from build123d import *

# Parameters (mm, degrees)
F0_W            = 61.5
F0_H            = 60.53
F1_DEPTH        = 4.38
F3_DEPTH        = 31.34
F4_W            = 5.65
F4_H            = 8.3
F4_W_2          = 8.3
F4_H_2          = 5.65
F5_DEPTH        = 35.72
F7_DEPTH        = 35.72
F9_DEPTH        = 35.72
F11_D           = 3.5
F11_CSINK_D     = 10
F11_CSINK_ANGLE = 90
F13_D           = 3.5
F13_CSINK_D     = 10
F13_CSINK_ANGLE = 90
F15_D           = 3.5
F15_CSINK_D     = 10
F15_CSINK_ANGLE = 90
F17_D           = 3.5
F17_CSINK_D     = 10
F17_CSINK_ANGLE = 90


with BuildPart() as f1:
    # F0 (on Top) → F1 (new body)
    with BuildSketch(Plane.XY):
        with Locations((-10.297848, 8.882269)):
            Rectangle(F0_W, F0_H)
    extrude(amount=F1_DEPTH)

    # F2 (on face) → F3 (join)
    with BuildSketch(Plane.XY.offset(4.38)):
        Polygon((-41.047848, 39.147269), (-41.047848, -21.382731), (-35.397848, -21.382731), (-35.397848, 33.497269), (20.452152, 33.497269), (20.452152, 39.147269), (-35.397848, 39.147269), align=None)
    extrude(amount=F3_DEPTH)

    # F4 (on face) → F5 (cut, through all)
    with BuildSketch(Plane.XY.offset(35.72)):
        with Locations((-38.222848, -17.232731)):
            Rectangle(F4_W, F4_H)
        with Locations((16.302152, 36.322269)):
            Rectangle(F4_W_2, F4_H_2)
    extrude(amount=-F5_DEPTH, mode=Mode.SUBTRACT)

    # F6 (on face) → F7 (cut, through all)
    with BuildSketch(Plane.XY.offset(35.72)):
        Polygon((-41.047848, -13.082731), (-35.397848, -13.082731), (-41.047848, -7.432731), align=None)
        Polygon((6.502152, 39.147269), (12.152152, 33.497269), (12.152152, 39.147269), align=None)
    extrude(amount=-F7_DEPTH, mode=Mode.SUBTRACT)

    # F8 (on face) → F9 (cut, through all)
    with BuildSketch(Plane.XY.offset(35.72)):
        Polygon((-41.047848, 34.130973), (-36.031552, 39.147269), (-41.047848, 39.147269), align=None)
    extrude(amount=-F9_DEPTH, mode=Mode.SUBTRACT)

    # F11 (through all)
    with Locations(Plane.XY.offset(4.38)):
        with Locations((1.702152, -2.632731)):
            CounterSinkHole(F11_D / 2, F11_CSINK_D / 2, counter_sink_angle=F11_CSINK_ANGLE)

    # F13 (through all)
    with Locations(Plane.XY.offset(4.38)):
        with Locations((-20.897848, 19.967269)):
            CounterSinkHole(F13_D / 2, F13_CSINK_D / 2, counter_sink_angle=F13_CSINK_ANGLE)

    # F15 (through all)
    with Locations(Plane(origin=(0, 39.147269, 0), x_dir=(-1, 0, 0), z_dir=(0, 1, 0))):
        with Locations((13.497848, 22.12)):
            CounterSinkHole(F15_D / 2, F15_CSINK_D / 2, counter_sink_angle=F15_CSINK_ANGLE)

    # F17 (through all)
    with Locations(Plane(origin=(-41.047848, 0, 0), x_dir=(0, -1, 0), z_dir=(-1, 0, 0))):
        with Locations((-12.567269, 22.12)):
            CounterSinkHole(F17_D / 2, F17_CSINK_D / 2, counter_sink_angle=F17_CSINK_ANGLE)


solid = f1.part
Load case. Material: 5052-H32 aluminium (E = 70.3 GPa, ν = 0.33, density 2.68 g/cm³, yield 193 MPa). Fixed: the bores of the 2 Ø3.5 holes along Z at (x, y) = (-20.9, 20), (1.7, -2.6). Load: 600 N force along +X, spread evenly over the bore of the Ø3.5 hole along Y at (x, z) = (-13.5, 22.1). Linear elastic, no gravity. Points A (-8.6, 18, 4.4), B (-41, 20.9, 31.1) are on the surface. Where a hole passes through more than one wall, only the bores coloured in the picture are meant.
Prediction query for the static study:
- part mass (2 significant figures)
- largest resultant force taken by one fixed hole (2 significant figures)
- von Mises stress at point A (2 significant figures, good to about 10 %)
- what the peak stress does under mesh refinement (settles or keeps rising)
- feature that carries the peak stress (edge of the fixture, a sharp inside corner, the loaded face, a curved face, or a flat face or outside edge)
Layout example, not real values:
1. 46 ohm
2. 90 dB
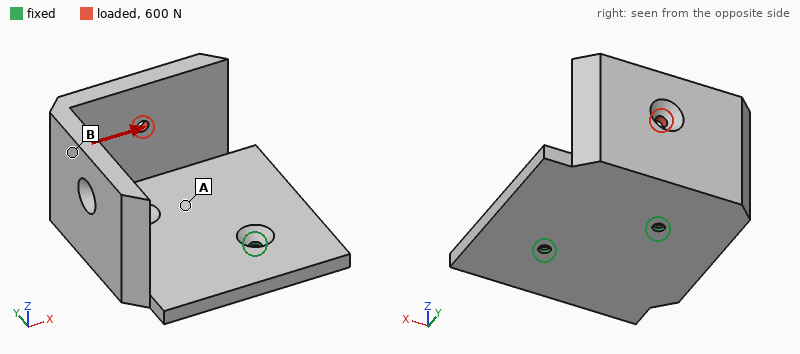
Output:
1. 84 g
2. 750 N
3. 37 MPa
4. keeps rising
5. edge of the fixture
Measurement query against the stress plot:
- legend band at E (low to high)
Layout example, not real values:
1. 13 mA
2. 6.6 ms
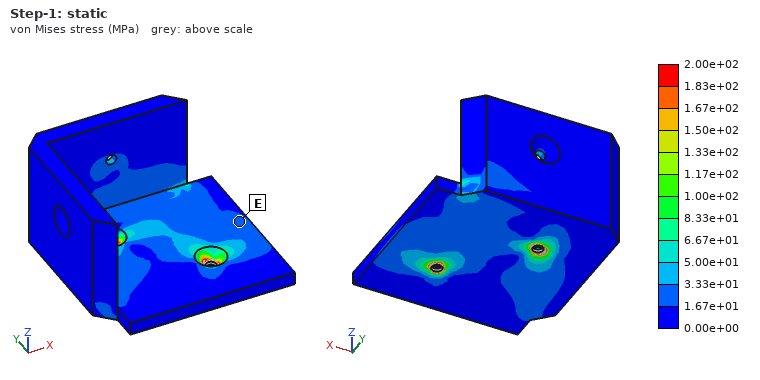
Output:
1. 1.67e+01 to 3.33e+01 MPa
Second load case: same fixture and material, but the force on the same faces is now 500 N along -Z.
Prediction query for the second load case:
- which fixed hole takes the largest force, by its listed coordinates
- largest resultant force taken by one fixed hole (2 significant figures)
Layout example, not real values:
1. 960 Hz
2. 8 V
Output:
1. (-20.9, 20)
2. 590 N
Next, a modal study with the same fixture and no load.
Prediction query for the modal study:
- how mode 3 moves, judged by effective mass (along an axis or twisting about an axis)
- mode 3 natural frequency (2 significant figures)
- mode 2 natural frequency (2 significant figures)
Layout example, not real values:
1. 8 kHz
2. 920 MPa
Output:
1. along Z
2. 3500 Hz
3. 1700 Hz
